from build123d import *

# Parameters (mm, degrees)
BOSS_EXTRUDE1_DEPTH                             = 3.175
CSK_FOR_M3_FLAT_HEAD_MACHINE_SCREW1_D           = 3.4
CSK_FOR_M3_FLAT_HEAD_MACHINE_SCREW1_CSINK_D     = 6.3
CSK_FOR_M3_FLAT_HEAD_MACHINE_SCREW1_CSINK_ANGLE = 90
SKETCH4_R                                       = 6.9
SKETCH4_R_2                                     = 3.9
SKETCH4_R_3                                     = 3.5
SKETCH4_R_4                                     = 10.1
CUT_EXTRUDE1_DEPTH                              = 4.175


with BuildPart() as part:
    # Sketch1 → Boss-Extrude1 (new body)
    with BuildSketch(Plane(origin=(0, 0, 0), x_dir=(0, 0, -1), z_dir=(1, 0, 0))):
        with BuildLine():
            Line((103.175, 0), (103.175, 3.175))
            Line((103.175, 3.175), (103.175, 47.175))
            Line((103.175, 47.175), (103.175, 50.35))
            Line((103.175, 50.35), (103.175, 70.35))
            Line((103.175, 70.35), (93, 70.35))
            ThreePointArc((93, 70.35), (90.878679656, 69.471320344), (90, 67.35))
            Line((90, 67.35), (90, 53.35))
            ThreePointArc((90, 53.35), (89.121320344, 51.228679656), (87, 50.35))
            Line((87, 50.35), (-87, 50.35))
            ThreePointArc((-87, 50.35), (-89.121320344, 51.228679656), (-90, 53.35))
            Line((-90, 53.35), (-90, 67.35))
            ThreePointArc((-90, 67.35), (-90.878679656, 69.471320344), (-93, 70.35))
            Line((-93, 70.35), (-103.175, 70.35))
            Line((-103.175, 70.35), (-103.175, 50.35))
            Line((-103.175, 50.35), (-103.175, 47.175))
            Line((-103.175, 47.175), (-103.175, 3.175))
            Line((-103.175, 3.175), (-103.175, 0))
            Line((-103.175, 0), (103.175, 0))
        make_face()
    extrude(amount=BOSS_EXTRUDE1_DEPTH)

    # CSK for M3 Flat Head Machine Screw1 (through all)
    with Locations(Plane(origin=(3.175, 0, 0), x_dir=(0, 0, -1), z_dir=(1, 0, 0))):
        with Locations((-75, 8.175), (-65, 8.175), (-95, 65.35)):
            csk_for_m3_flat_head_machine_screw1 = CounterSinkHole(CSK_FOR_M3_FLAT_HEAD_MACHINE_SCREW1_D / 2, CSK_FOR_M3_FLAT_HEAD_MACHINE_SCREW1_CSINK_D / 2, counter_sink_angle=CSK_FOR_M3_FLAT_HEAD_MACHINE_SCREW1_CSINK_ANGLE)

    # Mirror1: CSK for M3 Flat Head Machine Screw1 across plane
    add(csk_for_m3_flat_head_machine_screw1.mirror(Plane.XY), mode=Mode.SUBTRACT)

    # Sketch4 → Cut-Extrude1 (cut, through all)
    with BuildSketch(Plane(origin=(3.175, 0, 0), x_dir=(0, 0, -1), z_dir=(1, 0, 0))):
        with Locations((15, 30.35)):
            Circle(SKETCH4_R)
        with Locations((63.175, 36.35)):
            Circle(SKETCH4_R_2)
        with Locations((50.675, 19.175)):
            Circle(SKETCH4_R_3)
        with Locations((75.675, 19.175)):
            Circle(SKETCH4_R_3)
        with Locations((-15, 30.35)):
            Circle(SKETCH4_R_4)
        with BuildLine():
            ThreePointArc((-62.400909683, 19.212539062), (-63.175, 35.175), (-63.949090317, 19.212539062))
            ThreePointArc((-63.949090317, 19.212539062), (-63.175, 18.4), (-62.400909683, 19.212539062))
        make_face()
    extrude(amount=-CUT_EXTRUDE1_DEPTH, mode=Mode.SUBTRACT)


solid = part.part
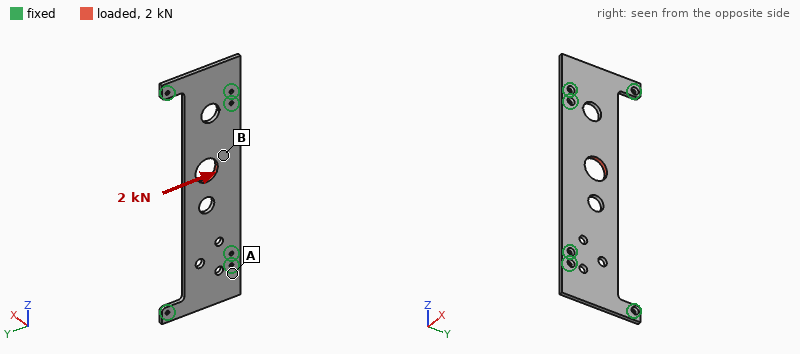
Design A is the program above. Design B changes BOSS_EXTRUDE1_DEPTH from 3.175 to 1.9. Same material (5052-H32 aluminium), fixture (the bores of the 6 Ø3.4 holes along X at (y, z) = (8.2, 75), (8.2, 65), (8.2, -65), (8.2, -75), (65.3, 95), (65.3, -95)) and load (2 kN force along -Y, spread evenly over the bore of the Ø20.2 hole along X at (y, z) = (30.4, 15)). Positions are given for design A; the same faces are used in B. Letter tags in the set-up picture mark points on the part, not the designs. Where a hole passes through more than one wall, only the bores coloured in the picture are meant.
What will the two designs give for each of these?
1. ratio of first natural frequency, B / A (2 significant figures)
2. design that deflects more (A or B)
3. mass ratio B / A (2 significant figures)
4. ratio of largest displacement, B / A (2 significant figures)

0.65
B
0.60
1.5
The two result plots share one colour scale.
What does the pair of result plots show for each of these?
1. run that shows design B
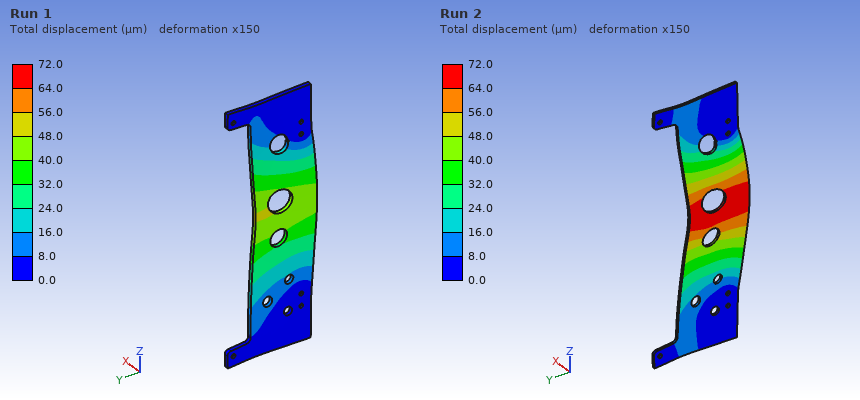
Run 2
